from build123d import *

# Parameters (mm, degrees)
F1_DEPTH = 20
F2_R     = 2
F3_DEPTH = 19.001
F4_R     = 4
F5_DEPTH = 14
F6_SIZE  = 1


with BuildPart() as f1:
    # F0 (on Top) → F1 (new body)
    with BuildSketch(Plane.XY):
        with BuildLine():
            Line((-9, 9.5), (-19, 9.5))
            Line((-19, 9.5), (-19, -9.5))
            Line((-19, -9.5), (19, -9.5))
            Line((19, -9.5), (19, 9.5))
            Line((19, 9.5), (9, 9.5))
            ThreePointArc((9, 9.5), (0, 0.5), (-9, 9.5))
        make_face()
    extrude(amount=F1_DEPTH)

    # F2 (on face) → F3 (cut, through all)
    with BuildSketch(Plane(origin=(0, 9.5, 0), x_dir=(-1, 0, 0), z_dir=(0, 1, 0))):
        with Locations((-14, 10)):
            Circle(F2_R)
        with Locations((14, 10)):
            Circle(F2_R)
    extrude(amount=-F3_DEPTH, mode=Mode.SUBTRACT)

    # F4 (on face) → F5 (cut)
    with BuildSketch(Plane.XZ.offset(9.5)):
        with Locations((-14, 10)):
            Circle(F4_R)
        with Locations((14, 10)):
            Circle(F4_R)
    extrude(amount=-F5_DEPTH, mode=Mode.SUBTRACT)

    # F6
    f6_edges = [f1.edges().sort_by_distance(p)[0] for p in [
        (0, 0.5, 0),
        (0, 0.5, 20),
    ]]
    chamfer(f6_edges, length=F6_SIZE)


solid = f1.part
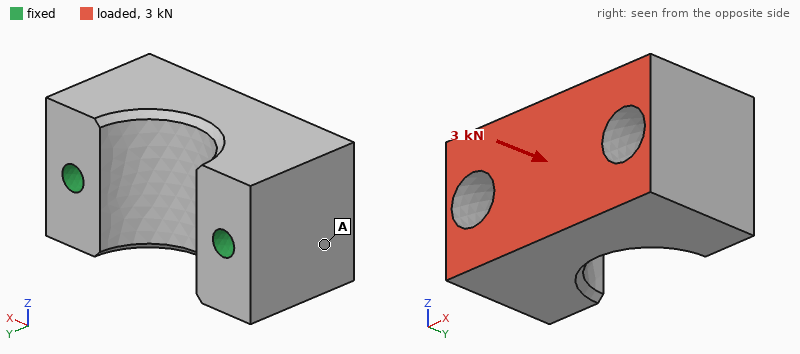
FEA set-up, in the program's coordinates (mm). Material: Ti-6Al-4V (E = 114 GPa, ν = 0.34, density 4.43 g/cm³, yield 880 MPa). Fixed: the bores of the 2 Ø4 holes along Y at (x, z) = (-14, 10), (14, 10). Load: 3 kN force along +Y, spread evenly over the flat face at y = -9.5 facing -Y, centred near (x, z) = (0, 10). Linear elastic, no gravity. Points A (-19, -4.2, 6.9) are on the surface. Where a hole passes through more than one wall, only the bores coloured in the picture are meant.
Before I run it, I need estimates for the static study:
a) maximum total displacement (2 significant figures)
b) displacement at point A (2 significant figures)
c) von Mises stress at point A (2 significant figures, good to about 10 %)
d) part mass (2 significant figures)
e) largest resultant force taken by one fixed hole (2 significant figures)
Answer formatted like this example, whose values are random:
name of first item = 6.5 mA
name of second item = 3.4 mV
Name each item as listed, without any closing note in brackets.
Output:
maximum total displacement = 3.3 µm
displacement at point A = 1.9 µm
von Mises stress at point A = 9.6 MPa
part mass = 46 g
largest resultant force taken by one fixed hole = 1.6 kN
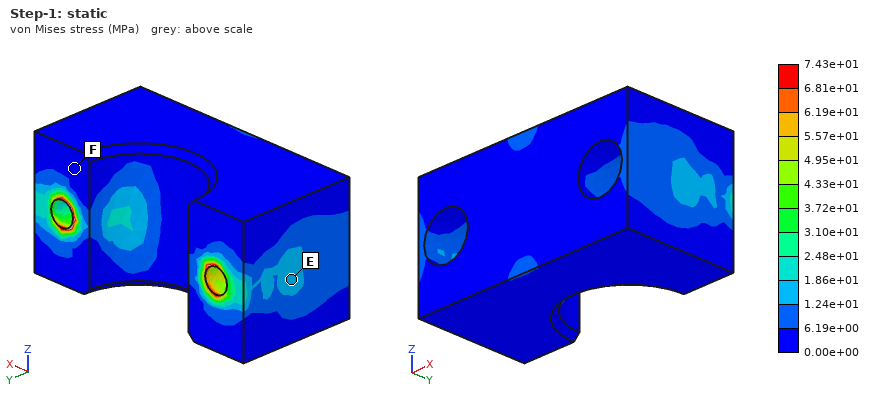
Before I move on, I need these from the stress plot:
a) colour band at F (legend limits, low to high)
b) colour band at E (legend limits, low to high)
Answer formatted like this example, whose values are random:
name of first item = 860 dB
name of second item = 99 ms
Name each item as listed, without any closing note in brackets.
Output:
colour band at F = 0.00e+00 to 6.19e+00 MPa
colour band at E = 1.24e+01 to 1.86e+01 MPa
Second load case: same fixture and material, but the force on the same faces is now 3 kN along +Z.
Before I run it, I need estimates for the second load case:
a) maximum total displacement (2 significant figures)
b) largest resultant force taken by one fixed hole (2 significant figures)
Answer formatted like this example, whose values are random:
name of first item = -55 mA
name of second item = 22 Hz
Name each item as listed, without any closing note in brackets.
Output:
maximum total displacement = 56 µm
largest resultant force taken by one fixed hole = 1.5 kN
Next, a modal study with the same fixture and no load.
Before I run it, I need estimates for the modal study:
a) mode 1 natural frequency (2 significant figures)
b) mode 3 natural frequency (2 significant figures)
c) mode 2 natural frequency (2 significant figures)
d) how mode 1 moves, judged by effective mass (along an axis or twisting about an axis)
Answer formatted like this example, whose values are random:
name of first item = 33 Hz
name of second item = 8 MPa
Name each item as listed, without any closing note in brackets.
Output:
mode 1 natural frequency = 8700 Hz
mode 3 natural frequency = 21 kHz
mode 2 natural frequency = 20 kHz
how mode 1 moves, judged by effective mass = along Z
